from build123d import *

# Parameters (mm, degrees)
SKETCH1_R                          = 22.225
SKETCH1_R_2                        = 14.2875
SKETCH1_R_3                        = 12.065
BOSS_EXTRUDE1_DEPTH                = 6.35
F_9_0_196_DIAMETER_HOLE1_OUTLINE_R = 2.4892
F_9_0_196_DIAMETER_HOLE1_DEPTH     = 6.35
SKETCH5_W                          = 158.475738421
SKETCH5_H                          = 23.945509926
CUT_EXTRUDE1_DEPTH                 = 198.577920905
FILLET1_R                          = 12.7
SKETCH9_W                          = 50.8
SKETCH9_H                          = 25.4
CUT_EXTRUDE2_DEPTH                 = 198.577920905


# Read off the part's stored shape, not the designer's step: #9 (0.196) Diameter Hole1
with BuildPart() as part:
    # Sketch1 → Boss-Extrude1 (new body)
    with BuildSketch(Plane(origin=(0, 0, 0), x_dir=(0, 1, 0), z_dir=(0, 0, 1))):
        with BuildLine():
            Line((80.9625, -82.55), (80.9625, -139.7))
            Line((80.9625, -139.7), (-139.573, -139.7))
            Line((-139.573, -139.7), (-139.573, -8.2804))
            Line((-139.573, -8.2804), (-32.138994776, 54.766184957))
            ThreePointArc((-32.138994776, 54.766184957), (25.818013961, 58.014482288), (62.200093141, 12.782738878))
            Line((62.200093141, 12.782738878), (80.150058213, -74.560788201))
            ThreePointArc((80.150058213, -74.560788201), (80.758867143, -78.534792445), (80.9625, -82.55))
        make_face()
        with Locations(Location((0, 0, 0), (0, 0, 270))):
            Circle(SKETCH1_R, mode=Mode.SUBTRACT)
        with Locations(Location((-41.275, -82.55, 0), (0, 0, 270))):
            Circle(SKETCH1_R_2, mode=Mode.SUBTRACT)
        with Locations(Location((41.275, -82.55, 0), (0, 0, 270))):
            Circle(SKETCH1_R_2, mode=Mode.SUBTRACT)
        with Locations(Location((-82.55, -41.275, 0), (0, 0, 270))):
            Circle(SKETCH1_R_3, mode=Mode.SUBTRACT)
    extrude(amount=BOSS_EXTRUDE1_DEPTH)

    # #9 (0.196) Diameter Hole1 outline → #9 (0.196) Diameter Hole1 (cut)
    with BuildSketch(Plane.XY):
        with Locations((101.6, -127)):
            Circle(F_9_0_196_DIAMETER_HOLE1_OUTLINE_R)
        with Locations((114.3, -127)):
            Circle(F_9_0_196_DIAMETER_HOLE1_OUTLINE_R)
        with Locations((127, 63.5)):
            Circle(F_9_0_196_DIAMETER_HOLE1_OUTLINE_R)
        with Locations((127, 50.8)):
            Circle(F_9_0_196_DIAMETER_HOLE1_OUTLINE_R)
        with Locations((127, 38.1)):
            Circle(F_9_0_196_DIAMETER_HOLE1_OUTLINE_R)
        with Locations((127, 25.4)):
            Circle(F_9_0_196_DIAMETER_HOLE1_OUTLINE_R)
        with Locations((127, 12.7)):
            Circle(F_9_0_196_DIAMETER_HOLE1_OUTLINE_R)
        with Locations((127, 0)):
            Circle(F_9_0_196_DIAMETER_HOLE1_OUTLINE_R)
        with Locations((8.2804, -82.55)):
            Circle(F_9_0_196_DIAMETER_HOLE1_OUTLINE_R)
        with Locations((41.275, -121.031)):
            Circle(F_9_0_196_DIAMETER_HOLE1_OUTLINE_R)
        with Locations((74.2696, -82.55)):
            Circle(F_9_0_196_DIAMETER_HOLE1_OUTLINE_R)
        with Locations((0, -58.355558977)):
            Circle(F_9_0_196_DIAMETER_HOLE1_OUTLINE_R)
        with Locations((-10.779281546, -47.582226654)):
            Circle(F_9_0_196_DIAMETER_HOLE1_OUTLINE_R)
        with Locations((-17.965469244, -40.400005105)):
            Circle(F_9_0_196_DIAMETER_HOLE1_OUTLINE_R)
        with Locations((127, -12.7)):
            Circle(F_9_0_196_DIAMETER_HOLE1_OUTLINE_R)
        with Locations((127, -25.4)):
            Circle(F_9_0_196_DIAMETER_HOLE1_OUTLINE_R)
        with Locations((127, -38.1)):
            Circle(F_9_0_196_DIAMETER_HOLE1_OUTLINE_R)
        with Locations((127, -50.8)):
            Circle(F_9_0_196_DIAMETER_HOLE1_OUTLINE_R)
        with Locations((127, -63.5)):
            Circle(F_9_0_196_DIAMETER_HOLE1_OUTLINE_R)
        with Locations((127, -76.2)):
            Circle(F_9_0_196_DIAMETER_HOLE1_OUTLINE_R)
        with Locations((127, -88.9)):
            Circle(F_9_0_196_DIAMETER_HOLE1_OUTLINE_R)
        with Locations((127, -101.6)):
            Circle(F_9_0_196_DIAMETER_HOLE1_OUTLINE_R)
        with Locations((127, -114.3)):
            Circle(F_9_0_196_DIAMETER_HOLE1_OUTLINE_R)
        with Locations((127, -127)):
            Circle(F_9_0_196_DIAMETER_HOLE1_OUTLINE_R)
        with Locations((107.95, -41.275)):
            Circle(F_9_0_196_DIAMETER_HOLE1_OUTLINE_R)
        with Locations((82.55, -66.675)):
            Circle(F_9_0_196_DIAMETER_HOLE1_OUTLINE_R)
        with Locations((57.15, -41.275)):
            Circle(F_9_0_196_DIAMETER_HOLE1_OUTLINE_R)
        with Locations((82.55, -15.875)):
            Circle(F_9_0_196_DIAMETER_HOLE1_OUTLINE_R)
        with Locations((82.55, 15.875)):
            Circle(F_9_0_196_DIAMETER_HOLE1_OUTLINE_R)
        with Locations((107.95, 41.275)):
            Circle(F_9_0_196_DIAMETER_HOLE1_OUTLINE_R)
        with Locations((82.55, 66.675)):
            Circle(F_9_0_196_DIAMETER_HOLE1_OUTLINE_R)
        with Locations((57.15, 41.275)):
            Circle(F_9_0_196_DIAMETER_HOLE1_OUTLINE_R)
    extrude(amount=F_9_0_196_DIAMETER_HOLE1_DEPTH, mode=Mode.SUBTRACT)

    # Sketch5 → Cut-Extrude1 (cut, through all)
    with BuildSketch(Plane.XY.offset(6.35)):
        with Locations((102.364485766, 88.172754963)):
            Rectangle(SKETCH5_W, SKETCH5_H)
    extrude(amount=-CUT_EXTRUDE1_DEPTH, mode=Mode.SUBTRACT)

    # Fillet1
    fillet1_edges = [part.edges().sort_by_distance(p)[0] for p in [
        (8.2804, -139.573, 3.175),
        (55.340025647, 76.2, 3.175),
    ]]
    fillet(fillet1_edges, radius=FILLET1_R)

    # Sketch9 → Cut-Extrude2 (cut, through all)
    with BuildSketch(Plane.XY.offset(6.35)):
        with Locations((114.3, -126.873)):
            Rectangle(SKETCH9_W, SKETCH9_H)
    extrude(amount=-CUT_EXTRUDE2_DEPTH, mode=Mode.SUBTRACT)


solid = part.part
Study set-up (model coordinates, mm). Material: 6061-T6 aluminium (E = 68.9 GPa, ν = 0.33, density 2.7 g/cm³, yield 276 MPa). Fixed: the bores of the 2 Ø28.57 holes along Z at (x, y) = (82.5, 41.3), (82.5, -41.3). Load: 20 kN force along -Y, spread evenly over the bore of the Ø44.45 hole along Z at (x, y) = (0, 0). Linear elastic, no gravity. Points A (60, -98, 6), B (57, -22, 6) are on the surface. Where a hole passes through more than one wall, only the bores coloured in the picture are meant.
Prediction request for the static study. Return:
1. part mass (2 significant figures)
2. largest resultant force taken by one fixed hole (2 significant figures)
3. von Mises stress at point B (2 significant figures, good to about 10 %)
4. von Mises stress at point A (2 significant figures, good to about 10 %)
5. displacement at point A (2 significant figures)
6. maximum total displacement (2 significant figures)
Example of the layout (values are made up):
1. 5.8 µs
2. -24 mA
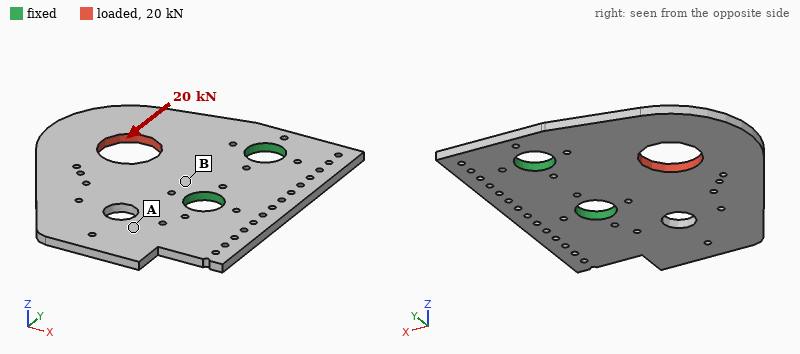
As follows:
1. 550 g
2. 18 kN
3. 54 MPa
4. 17 MPa
5. 0.063 mm
6. 0.16 mm
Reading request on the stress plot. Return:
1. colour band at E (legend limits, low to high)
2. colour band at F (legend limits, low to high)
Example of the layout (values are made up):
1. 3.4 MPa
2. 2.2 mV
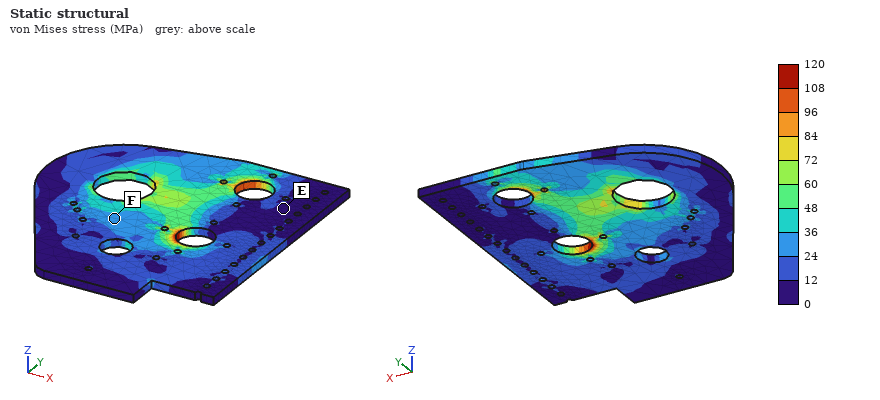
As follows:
1. 0 to 12 MPa
2. 24 to 36 MPa
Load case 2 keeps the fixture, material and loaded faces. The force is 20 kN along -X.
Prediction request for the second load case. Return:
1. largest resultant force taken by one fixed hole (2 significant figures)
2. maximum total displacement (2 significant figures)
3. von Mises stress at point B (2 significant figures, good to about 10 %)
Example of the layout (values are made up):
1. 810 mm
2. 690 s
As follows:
1. 10 kN
2. 53 µm
3. 25 MPa
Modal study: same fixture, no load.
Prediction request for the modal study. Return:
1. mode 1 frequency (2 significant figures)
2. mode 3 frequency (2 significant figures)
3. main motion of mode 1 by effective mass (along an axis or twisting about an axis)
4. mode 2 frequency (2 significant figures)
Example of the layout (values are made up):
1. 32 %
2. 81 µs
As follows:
1. 360 Hz
2. 940 Hz
3. along Z
4. 560 Hz
